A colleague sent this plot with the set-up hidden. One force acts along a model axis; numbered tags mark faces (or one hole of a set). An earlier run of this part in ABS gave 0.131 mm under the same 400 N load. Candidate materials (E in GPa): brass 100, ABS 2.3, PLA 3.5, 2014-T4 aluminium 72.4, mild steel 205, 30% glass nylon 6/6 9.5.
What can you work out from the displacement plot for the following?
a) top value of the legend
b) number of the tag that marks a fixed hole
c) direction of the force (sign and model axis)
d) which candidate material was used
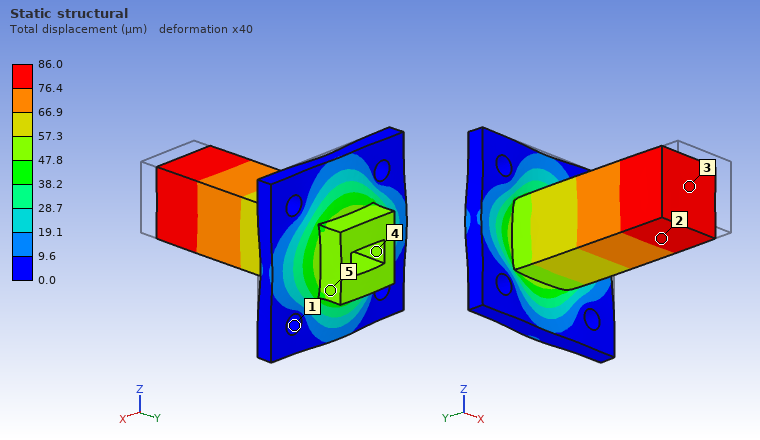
86.0 µm
1
+Y
PLA
